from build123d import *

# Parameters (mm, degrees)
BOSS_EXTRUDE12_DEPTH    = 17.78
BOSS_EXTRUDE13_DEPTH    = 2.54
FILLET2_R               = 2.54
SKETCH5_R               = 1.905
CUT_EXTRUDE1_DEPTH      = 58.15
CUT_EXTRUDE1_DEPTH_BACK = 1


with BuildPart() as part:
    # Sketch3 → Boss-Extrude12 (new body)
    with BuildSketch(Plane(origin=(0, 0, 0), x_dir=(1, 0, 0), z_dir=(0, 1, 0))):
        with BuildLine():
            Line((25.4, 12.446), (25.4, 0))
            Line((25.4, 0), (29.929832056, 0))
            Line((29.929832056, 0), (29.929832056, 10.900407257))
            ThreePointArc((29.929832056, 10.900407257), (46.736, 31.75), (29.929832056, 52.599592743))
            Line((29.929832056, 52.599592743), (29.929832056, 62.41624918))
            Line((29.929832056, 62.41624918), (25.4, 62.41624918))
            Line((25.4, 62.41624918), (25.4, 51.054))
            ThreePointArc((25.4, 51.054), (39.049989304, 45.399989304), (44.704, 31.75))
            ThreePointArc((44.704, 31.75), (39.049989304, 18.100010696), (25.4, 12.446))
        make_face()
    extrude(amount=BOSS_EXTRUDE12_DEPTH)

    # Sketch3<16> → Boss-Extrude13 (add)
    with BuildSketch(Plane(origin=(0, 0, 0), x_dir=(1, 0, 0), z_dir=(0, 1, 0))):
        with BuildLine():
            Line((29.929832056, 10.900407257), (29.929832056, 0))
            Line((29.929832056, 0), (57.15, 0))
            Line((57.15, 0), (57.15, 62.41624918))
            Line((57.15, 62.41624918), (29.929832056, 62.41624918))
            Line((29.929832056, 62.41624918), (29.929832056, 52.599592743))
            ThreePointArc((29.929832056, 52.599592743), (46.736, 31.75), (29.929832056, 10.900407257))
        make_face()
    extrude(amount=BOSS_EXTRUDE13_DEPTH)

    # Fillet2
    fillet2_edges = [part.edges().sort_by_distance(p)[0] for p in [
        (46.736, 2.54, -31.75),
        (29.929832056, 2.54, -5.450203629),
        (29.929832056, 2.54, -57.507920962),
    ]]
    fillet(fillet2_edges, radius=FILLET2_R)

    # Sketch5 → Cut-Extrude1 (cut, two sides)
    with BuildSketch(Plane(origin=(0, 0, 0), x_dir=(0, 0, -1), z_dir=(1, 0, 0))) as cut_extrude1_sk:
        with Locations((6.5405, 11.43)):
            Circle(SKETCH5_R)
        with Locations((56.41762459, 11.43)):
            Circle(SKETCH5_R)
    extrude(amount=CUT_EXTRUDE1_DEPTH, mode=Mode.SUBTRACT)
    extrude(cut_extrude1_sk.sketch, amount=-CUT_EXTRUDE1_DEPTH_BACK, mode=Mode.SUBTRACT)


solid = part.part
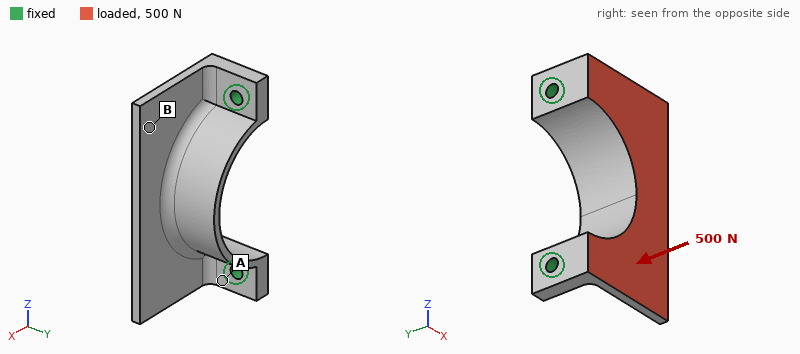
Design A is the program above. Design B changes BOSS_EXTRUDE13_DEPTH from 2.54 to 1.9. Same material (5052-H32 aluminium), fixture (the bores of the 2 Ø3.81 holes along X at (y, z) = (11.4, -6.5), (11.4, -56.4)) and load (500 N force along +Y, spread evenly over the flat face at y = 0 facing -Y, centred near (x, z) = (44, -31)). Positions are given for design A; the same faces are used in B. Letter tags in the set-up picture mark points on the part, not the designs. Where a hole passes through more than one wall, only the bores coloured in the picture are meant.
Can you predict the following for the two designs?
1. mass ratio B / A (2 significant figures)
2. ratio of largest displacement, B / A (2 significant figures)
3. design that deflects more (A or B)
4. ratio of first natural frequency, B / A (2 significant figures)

0.89
1.6
B
1.00
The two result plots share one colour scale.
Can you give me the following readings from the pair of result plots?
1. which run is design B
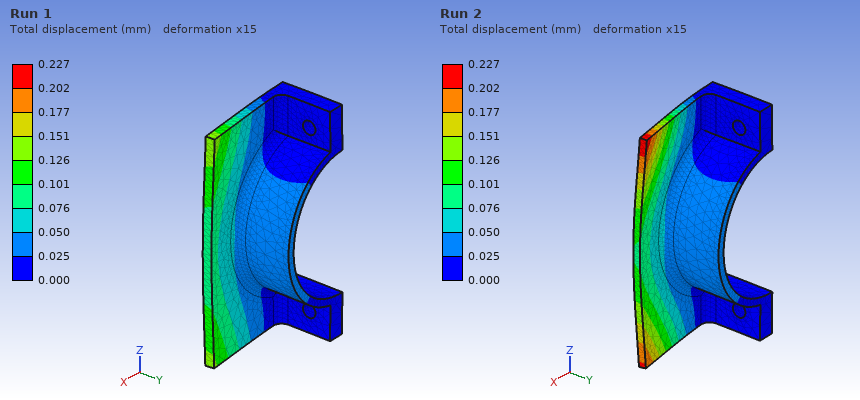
Run 2
